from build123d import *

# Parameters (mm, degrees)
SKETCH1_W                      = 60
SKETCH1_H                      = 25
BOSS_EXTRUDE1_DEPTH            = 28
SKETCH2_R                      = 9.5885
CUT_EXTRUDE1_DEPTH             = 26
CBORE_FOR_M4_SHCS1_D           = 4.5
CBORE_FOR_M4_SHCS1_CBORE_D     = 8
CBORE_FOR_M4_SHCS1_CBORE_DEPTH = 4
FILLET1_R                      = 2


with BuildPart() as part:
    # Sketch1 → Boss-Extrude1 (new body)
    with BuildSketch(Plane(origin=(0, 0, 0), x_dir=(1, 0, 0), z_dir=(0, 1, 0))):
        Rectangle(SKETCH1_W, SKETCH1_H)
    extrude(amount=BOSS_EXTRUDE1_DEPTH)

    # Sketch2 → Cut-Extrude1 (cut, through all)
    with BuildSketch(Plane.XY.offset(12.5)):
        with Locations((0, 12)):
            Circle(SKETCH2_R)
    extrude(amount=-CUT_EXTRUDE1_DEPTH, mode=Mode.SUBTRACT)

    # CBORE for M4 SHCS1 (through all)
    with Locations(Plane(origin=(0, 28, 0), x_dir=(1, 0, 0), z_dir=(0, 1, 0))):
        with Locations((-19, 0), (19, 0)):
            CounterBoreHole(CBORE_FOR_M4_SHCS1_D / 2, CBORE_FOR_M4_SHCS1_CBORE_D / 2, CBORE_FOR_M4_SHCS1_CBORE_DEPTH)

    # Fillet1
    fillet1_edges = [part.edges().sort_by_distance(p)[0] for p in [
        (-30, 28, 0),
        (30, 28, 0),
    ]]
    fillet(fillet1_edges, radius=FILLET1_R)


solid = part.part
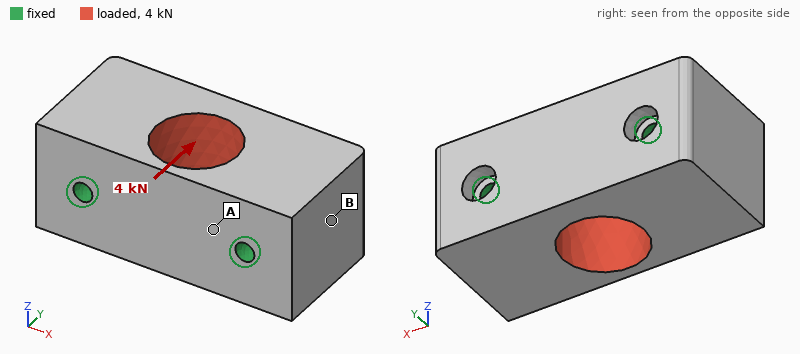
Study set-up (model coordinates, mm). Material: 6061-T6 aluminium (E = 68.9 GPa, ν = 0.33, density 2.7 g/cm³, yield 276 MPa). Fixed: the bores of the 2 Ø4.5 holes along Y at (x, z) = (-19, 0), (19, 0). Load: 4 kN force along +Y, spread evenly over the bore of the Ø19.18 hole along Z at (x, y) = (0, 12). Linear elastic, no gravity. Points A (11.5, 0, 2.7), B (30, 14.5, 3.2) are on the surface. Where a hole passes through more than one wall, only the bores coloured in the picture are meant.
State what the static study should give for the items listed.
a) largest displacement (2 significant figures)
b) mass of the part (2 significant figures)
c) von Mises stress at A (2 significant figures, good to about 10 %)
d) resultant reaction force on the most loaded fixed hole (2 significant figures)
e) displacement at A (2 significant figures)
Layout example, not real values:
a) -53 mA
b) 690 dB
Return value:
a) 5.7 µm
b) 91 g
c) 4.4 MPa
d) 2.0 kN
e) 1.7 µm
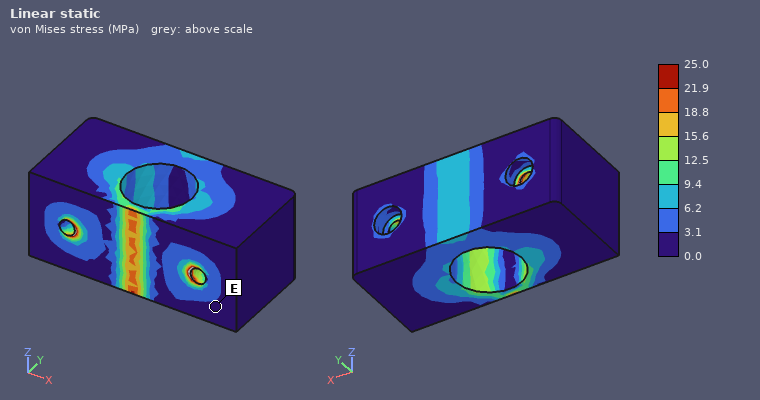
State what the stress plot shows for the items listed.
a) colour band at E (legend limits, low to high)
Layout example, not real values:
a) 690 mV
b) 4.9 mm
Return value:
a) 0.0 to 3.1 MPa
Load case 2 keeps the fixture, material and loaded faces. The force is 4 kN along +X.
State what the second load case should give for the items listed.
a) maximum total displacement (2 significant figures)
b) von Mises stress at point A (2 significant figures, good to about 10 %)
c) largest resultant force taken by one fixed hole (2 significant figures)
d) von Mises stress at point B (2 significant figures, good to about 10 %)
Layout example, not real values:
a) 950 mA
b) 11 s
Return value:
a) 1.4 µm
b) 5.7 MPa
c) 2.0 kN
d) 1.9 MPa
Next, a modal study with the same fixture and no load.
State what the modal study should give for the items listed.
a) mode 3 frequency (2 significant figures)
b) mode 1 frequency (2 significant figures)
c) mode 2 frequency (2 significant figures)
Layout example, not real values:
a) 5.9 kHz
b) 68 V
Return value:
a) 31 kHz
b) 23 kHz
c) 30 kHz
